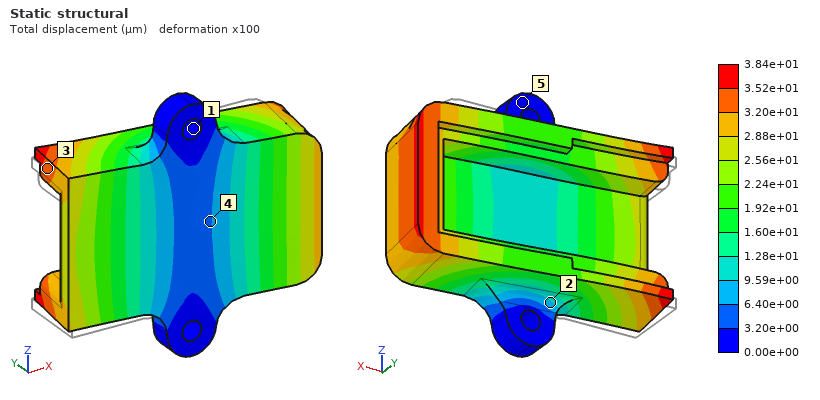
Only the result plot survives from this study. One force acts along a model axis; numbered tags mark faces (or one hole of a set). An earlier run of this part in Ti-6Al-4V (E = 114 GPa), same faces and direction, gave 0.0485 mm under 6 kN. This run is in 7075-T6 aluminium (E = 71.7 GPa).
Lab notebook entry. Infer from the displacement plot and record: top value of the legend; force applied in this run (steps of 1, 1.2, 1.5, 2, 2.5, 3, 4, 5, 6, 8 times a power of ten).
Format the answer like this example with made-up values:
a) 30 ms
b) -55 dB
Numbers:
a) 3.84e+01 µm
b) 3 kN
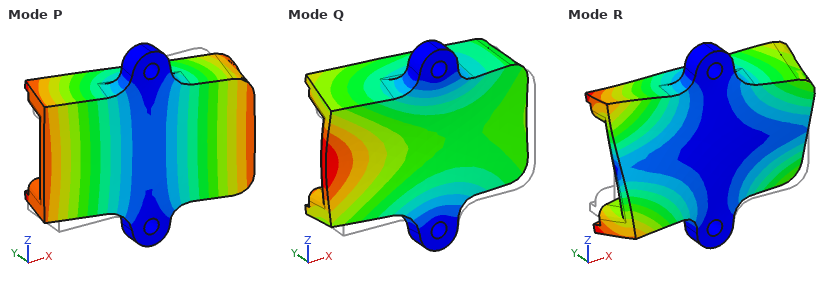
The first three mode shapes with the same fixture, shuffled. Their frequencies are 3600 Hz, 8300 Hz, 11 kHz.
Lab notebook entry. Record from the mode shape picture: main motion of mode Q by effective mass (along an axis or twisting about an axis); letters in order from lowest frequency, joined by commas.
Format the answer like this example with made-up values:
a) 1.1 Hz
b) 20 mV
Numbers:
a) along Y
b) P, Q, R
